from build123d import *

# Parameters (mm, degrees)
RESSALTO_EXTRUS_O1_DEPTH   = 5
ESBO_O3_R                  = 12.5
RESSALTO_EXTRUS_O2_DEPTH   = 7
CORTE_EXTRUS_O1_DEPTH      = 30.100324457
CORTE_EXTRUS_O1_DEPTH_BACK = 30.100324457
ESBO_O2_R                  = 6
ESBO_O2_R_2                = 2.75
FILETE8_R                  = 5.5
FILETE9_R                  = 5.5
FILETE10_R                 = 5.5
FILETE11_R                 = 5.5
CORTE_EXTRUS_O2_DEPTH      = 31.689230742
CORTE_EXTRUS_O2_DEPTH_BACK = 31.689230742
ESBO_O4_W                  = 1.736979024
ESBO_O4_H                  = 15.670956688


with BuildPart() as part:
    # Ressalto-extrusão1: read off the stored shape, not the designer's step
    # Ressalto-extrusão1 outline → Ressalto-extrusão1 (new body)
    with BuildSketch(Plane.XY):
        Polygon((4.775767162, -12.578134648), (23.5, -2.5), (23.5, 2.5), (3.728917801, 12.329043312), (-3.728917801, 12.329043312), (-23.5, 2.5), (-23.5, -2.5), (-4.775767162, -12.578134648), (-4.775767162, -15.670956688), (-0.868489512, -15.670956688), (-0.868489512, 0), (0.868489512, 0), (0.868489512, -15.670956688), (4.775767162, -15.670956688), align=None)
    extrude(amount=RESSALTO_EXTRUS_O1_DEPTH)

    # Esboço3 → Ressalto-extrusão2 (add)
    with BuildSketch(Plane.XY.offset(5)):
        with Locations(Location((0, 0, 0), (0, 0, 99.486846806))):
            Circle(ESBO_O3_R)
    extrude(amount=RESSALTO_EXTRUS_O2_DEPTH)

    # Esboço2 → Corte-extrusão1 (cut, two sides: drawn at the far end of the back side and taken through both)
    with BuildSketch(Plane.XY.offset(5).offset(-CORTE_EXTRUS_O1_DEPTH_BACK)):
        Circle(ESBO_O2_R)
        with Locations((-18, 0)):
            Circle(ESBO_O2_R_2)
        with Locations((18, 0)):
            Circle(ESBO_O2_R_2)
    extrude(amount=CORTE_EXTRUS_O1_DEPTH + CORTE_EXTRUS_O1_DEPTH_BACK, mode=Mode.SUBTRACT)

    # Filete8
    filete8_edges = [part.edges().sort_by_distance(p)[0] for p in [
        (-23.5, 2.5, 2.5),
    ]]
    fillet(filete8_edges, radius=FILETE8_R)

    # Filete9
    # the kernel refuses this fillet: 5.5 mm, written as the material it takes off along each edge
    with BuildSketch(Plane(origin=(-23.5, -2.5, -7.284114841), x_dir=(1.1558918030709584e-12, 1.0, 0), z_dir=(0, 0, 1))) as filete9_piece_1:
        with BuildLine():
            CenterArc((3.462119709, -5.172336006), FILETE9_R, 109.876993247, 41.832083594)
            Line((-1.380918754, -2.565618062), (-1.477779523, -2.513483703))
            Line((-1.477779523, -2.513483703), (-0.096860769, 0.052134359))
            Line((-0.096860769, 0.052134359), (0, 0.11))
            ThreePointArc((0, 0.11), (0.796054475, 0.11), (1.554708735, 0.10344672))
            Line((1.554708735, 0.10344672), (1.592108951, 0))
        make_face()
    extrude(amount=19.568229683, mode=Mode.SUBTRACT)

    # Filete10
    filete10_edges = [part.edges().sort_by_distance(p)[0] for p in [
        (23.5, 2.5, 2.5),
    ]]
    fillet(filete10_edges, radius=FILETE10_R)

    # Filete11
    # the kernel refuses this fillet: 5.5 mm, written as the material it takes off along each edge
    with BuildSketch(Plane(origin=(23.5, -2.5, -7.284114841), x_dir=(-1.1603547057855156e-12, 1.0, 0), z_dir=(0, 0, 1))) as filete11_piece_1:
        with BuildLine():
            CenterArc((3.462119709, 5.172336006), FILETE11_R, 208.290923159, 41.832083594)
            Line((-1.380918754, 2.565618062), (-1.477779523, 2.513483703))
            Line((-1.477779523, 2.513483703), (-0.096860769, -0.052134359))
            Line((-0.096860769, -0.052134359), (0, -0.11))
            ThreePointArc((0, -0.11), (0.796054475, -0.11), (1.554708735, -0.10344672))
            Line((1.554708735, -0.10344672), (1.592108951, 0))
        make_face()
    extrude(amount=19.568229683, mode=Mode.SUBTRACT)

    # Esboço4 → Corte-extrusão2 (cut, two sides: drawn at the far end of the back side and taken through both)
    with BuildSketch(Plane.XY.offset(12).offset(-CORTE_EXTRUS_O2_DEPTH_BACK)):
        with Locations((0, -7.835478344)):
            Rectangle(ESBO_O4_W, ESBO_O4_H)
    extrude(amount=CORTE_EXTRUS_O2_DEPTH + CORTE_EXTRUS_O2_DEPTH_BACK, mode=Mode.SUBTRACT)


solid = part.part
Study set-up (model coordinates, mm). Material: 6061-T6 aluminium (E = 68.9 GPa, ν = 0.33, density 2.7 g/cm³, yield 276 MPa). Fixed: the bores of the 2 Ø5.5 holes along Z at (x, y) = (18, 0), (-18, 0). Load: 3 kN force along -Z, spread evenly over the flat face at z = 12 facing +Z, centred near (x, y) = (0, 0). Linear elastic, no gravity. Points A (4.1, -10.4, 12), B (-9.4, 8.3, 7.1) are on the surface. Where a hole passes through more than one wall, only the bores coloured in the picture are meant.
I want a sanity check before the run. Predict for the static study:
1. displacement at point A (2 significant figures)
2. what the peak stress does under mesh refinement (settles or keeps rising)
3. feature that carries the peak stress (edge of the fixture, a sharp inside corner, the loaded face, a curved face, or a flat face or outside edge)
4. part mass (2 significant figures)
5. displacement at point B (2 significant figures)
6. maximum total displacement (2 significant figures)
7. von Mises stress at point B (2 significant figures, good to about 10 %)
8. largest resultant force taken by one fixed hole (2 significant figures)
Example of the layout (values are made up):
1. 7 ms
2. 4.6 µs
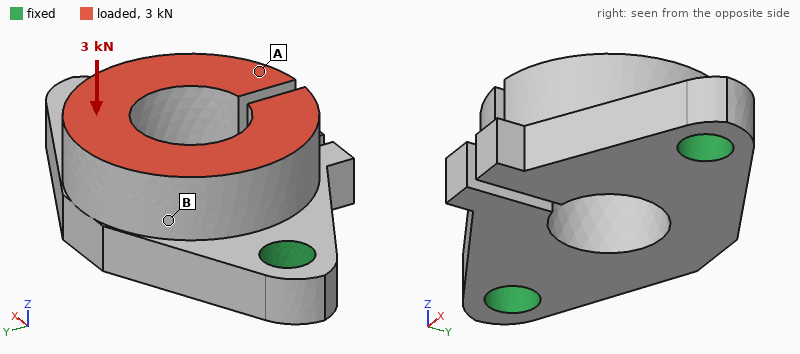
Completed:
1. 45 µm
2. keeps rising
3. edge of the fixture
4. 15 g
5. 20 µm
6. 54 µm
7. 57 MPa
8. 1.6 kN
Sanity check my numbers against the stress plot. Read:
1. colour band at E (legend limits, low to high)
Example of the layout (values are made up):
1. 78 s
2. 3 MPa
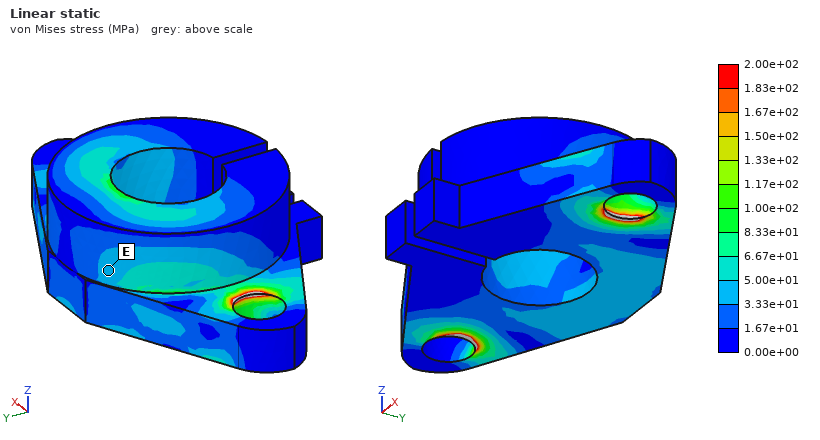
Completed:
1. 3.33e+01 to 5.00e+01 MPa
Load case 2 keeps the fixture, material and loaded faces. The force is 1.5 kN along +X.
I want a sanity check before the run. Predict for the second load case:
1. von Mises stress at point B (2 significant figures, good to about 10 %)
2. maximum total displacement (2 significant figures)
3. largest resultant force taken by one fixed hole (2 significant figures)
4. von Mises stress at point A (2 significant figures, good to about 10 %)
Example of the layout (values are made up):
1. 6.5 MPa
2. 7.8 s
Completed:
1. 10 MPa
2. 33 µm
3. 850 N
4. 9.4 MPa
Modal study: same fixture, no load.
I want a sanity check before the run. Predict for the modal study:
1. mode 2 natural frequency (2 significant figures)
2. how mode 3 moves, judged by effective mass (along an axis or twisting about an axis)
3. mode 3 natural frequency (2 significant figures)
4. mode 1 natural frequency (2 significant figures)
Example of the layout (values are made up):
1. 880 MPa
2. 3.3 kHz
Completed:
1. 12 kHz
2. along Z
3. 13 kHz
4. 11 kHz
